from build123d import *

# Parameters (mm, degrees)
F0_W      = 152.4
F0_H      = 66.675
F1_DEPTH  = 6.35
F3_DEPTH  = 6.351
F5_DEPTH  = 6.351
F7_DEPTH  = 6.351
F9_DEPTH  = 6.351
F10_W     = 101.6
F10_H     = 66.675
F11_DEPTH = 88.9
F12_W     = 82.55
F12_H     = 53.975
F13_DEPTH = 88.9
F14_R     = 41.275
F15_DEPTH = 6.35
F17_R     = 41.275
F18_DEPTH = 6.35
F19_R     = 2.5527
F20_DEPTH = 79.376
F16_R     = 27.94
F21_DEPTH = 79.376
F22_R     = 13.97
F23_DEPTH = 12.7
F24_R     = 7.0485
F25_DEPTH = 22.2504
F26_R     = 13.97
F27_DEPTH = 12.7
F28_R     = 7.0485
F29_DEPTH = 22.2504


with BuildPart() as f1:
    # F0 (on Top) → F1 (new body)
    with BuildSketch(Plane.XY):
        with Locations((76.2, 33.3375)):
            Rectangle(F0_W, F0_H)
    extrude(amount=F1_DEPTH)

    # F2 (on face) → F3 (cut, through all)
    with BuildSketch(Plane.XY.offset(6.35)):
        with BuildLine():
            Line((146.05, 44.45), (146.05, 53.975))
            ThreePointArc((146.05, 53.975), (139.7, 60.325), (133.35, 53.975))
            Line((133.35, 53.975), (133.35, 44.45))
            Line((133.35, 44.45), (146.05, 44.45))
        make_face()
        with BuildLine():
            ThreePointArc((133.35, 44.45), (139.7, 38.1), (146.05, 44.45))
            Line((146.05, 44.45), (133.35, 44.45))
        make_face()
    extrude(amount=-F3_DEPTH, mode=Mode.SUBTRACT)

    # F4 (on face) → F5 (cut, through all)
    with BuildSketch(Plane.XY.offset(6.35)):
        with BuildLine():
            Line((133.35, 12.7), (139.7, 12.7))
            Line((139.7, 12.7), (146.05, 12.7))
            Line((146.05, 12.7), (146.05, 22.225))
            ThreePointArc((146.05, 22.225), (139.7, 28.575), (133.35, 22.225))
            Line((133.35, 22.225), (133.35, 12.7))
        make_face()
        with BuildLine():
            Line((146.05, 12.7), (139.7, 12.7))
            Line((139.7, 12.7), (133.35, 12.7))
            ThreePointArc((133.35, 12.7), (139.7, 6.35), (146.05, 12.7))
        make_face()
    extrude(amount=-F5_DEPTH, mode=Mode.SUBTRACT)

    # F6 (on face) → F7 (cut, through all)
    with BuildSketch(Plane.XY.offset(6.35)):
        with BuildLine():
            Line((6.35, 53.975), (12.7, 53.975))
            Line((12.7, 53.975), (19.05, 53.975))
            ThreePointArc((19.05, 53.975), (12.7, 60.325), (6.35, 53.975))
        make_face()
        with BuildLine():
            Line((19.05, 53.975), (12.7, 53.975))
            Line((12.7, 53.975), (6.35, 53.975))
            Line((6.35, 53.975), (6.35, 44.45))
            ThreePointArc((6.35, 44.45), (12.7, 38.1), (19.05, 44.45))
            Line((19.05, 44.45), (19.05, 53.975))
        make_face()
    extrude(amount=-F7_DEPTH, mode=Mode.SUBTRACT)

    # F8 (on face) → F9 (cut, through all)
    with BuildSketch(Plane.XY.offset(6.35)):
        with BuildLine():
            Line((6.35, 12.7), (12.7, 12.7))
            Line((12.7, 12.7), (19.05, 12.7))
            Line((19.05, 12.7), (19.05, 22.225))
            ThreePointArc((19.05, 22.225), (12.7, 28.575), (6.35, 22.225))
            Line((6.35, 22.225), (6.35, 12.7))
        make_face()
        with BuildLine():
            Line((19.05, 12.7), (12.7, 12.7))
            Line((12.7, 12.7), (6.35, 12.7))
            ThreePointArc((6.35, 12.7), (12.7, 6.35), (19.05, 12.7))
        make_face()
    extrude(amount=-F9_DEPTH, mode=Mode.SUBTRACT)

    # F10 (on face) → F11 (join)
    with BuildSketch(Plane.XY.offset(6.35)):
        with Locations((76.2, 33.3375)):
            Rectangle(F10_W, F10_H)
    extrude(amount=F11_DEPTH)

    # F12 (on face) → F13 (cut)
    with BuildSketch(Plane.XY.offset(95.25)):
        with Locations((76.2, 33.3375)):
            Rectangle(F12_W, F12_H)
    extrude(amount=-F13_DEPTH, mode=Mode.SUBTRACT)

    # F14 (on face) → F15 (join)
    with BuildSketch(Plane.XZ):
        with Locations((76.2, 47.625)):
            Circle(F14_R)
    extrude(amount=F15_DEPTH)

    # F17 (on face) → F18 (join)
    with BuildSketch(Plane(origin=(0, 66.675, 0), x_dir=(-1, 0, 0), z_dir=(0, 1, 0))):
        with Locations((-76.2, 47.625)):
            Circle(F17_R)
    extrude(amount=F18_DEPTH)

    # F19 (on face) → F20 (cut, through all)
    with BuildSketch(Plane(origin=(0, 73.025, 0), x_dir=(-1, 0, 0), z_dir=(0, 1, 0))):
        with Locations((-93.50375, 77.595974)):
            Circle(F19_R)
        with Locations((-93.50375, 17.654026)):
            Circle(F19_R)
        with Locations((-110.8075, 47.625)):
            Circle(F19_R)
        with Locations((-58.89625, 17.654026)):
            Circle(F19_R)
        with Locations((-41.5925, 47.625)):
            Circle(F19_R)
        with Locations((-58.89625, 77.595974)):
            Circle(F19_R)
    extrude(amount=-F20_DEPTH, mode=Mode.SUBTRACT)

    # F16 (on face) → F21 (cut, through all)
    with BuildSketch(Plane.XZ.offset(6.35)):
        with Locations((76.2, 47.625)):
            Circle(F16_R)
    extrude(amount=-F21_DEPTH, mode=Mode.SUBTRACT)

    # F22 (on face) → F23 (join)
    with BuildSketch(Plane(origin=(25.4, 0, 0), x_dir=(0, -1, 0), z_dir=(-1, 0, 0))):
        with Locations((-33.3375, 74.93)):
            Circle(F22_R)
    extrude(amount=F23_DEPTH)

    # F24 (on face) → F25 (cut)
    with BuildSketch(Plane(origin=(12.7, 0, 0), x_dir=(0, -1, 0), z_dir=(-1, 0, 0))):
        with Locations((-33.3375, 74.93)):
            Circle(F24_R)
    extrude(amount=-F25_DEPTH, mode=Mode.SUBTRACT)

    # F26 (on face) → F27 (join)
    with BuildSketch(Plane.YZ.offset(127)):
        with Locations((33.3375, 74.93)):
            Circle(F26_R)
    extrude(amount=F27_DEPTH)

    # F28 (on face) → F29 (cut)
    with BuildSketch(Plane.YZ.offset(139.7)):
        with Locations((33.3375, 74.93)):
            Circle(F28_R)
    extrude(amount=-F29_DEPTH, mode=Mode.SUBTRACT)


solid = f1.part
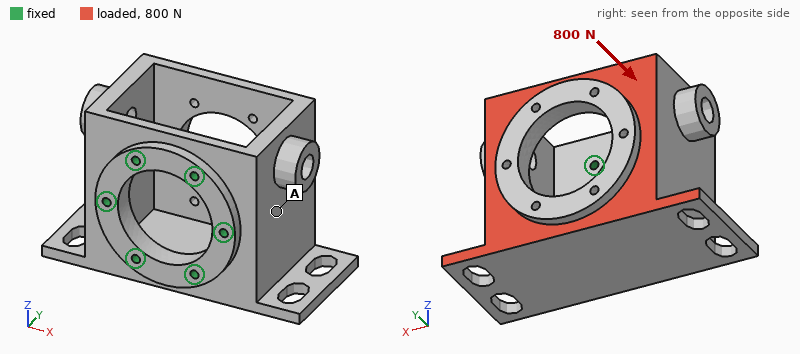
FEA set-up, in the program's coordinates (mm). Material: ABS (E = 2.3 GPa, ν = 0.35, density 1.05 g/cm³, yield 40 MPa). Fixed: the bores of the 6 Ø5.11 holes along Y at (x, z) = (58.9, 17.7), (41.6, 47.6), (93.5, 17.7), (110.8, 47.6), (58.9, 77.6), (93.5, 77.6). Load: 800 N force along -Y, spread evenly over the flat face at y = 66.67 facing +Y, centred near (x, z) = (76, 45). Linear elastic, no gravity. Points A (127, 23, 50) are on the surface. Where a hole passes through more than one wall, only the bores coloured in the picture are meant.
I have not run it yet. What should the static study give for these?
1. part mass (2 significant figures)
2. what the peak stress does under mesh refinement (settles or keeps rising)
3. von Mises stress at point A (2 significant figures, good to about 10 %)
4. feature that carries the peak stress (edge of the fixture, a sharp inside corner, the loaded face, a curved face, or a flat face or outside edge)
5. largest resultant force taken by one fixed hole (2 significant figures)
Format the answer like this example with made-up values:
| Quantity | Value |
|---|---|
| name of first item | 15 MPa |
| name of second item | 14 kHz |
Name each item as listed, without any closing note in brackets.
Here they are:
| Quantity | Value |
|---|---|
| part mass | 290 g |
| what the peak stress does under mesh refinement | keeps rising |
| von Mises stress at point A | 0.58 MPa |
| feature that carries the peak stress | edge of the fixture |
| largest resultant force taken by one fixed hole | 290 N |
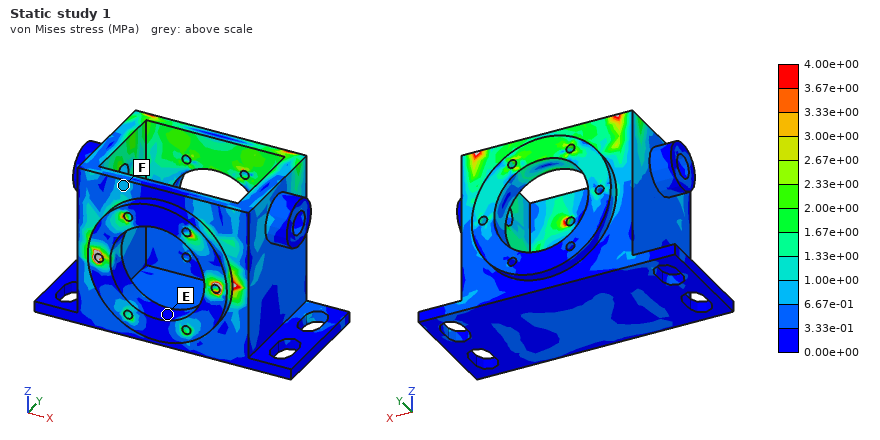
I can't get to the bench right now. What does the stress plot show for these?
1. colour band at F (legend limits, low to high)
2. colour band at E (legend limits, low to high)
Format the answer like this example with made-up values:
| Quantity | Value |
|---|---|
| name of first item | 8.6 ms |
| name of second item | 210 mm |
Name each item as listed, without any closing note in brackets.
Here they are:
| Quantity | Value |
|---|---|
| colour band at F | 6.67e-01 to 1.00e+00 MPa |
| colour band at E | 0.00e+00 to 3.33e-01 MPa |
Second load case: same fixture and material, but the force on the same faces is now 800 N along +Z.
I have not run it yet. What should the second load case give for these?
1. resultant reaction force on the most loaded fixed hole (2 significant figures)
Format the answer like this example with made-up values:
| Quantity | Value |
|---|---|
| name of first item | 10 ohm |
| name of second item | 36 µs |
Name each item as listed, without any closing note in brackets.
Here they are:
| Quantity | Value |
|---|---|
| resultant reaction force on the most loaded fixed hole | 490 N |
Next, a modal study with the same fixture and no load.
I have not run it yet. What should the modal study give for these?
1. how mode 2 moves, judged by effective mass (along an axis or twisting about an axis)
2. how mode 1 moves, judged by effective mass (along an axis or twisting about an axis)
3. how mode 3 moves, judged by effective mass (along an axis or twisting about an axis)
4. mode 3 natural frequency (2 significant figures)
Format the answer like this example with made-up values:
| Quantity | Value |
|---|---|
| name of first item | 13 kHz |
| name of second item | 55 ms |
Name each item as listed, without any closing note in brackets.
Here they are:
| Quantity | Value |
|---|---|
| how mode 2 moves, judged by effective mass | along Z |
| how mode 1 moves, judged by effective mass | along X |
| how mode 3 moves, judged by effective mass | along Y |
| mode 3 natural frequency | 1200 Hz |
